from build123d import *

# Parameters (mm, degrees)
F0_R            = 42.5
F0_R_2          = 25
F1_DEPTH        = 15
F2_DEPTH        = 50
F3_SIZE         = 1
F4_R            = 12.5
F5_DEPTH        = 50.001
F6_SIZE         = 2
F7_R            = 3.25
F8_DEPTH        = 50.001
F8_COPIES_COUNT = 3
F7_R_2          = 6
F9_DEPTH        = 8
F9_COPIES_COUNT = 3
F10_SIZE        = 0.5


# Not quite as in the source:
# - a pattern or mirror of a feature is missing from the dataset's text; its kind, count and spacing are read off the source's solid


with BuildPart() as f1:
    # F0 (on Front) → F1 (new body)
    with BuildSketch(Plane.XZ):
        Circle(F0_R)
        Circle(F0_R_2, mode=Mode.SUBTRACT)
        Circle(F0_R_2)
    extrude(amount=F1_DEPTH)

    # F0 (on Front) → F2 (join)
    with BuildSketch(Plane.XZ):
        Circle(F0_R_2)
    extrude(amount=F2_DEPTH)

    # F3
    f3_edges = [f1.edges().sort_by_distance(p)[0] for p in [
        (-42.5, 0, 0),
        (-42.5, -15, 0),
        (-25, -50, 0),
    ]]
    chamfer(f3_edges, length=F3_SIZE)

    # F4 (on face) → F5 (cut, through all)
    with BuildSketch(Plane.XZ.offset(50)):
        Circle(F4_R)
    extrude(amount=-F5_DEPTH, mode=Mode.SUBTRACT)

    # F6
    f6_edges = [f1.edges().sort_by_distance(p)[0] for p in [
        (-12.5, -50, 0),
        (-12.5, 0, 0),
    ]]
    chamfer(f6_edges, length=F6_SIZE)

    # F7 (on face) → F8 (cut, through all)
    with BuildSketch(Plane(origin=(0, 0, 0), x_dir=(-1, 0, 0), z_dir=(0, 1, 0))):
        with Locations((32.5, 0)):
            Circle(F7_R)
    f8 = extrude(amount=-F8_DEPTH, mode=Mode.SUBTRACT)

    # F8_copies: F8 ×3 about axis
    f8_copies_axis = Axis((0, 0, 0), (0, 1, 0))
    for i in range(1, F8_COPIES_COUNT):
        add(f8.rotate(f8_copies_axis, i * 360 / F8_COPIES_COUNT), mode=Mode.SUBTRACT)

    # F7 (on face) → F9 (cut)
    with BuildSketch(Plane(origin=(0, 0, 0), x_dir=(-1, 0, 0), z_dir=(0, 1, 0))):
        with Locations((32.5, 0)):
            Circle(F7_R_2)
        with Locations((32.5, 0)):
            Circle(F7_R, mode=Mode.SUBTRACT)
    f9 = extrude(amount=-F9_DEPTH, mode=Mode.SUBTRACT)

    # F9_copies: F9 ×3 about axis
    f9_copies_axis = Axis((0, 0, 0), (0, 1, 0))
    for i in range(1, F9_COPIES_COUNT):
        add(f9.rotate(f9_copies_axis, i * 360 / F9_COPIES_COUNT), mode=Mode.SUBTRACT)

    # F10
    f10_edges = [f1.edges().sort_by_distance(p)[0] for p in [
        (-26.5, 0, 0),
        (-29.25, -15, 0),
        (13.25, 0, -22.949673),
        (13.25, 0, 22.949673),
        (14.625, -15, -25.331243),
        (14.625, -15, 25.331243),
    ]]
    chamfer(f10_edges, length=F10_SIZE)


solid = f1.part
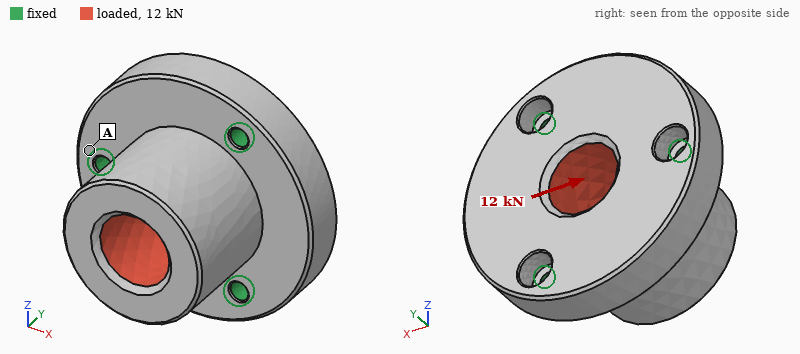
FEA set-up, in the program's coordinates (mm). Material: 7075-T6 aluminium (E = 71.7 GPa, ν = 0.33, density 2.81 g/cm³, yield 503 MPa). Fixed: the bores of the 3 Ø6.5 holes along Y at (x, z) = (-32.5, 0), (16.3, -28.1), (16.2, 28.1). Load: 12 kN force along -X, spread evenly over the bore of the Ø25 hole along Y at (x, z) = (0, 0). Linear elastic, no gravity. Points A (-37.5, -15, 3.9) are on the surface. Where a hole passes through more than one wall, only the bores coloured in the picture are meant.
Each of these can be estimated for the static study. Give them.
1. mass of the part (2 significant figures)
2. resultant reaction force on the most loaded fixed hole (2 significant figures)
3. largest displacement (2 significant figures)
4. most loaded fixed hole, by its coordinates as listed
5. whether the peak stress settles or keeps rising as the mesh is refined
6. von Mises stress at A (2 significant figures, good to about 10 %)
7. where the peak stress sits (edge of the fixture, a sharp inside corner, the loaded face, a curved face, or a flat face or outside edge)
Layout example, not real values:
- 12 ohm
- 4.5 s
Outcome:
- 350 g
- 5.1 kN
- 29 µm
- (-32.5, 0)
- keeps rising
- 9.5 MPa
- edge of the fixture
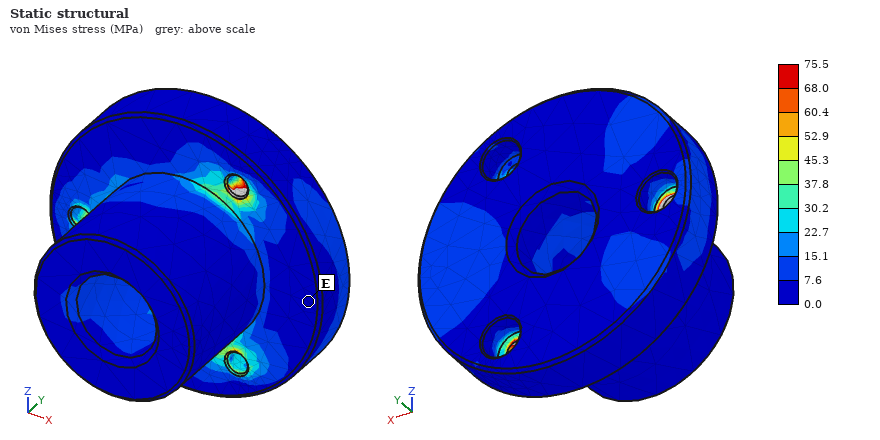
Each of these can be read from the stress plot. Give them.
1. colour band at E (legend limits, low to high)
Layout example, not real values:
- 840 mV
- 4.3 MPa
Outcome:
- 0.0 to 7.6 MPa
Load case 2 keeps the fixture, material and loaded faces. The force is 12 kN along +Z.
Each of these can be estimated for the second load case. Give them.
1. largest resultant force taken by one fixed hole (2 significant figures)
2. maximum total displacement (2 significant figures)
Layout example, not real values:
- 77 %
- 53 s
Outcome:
- 4.9 kN
- 28 µm
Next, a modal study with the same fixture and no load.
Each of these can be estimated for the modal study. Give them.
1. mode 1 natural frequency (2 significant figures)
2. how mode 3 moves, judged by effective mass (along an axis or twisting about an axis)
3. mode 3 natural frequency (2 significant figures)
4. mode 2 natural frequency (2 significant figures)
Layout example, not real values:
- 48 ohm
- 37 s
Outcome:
- 7200 Hz
- along Y
- 9400 Hz
- 7200 Hz
